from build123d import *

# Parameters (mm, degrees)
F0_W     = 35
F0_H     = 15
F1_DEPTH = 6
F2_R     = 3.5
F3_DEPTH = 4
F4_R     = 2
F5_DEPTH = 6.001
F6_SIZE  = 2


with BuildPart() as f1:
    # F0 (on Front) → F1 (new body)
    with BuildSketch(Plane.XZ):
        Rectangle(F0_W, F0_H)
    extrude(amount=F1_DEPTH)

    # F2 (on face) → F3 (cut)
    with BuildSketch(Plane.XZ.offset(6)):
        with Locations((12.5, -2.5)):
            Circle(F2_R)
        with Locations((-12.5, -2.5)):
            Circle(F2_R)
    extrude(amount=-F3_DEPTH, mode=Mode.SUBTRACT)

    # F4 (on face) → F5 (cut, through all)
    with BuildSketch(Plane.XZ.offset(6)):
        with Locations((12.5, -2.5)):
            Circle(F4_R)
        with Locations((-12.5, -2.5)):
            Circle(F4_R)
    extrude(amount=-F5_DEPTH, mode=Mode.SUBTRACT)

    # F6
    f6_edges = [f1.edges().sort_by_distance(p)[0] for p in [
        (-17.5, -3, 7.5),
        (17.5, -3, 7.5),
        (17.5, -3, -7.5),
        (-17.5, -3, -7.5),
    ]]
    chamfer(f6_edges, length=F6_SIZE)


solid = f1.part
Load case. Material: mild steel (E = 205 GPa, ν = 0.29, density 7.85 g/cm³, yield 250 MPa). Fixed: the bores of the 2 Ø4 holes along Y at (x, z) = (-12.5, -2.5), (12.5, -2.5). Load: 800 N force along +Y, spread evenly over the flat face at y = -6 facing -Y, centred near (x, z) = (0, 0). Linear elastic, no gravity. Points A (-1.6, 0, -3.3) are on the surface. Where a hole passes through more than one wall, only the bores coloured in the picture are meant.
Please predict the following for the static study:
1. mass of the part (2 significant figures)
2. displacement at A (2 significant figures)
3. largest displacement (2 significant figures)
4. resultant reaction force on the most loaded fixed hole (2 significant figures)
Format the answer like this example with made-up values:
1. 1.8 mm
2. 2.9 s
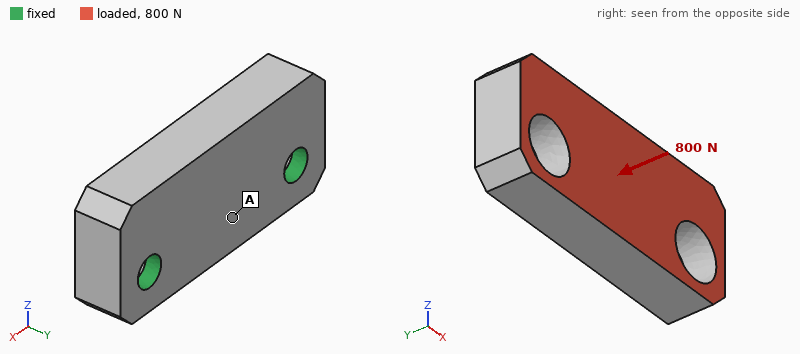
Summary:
1. 22 g
2. 1.3 µm
3. 6.0 µm
4. 430 N
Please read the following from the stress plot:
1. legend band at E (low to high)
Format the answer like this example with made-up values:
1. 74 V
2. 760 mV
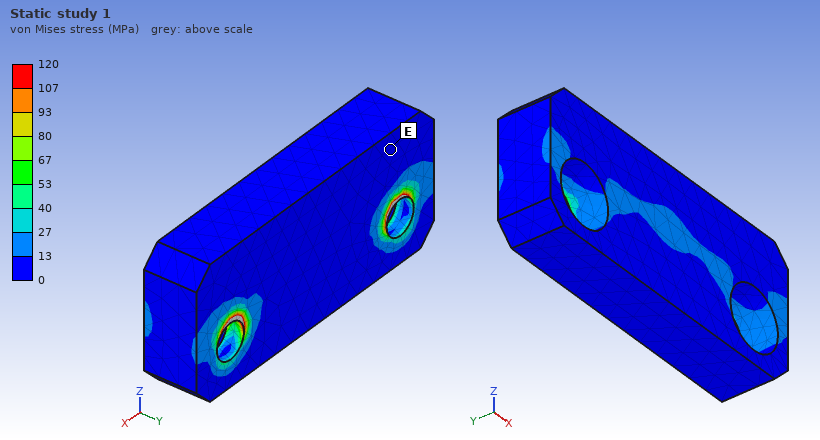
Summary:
1. 0 to 13 MPa
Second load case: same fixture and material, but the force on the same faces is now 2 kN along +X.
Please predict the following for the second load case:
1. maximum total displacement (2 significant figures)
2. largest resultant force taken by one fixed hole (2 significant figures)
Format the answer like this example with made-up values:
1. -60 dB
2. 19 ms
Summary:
1. 3.1 µm
2. 1.1 kN
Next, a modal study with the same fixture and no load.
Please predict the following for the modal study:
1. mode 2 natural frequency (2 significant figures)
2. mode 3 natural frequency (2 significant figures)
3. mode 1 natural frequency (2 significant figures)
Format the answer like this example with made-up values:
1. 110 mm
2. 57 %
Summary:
1. 29 kHz
2. 29 kHz
3. 14 kHz
